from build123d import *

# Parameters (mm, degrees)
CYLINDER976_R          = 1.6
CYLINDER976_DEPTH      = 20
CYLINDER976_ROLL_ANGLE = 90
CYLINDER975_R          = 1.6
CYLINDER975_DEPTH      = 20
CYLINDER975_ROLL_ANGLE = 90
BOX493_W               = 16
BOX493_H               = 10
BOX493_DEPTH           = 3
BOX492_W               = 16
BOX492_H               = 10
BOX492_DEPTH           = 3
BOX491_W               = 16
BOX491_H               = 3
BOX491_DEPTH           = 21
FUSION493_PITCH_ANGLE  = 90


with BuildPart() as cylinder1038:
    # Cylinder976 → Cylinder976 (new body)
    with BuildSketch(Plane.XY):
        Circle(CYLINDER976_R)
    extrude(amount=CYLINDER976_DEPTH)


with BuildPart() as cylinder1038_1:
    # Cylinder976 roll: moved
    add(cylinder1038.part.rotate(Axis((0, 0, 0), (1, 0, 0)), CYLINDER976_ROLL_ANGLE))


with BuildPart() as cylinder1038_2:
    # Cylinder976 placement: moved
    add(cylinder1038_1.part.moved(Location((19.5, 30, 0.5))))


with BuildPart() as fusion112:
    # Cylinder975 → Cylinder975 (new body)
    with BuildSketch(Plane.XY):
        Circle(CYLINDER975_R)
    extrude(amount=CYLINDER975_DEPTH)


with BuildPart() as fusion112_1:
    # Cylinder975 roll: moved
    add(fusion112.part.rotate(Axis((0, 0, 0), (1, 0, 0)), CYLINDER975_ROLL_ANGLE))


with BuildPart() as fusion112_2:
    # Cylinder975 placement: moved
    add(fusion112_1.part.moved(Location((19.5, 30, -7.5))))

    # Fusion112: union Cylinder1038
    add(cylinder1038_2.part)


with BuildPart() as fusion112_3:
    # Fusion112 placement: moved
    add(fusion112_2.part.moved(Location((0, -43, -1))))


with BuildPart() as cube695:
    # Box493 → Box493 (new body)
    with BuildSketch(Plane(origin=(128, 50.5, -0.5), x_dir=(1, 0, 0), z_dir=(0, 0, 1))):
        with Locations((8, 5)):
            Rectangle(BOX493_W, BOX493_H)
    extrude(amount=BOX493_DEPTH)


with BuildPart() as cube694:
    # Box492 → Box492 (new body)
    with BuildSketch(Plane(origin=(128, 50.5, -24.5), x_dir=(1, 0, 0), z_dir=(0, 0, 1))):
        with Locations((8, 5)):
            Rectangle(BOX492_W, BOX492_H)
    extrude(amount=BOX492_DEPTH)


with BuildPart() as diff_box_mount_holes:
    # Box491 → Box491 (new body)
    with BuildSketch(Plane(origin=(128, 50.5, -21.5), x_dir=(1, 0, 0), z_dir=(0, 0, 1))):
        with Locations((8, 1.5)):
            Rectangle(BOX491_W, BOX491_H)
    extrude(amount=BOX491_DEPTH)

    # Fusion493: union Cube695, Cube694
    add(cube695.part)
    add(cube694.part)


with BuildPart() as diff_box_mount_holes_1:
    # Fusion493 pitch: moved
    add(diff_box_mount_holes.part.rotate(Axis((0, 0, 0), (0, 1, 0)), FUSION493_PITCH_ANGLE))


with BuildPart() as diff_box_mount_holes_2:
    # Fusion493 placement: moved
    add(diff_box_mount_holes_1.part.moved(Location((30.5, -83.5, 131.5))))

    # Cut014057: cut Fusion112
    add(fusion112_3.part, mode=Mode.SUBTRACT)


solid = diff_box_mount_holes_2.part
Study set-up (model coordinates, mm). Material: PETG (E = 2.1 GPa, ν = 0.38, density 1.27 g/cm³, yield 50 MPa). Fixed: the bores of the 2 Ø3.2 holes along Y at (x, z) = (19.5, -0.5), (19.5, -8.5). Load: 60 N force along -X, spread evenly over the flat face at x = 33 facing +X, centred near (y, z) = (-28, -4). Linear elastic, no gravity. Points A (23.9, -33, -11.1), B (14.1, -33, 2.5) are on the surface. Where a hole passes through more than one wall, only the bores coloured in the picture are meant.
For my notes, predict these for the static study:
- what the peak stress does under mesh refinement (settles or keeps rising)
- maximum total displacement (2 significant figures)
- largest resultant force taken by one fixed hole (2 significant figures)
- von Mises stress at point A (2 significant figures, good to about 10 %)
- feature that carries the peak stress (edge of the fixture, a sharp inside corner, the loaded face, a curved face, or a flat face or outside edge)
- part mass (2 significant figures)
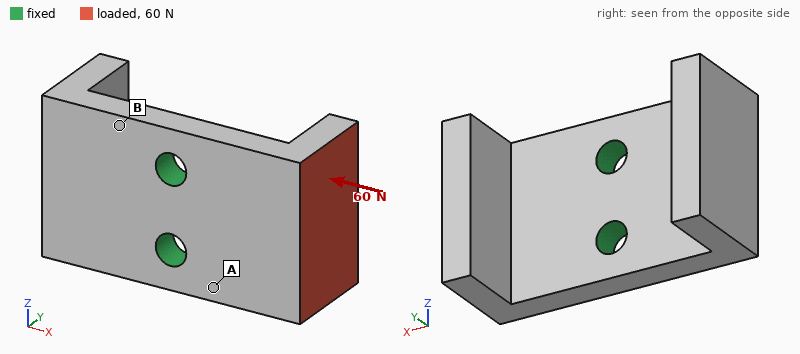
keeps rising
0.35 mm
31 N
7.3 MPa
edge of the fixture
2.4 g
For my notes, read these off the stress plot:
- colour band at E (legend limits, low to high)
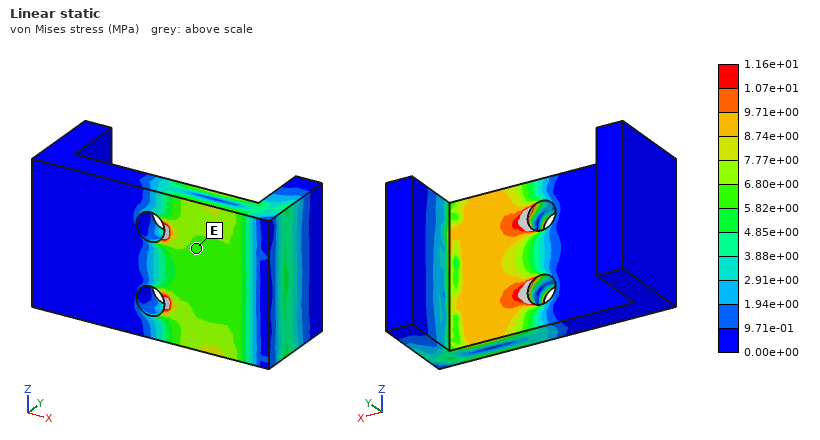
5.82e+00 to 6.80e+00 MPa
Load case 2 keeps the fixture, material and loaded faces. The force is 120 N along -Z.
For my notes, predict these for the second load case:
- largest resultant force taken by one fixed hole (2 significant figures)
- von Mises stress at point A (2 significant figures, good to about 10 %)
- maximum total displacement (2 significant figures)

170 N
13 MPa
0.35 mm
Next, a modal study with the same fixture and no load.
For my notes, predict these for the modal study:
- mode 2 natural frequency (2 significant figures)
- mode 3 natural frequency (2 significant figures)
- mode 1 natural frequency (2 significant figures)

2100 Hz
3600 Hz
2100 Hz
